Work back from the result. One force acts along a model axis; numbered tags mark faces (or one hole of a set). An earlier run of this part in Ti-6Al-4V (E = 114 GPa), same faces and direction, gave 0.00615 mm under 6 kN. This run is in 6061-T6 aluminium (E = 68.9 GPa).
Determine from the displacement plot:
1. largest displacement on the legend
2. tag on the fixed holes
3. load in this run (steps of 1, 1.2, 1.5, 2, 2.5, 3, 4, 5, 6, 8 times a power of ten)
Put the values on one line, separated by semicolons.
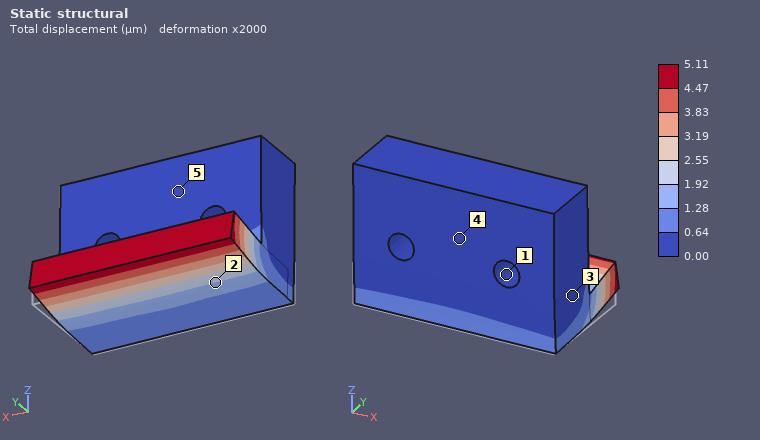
5.11 µm; 1; 3 kN
